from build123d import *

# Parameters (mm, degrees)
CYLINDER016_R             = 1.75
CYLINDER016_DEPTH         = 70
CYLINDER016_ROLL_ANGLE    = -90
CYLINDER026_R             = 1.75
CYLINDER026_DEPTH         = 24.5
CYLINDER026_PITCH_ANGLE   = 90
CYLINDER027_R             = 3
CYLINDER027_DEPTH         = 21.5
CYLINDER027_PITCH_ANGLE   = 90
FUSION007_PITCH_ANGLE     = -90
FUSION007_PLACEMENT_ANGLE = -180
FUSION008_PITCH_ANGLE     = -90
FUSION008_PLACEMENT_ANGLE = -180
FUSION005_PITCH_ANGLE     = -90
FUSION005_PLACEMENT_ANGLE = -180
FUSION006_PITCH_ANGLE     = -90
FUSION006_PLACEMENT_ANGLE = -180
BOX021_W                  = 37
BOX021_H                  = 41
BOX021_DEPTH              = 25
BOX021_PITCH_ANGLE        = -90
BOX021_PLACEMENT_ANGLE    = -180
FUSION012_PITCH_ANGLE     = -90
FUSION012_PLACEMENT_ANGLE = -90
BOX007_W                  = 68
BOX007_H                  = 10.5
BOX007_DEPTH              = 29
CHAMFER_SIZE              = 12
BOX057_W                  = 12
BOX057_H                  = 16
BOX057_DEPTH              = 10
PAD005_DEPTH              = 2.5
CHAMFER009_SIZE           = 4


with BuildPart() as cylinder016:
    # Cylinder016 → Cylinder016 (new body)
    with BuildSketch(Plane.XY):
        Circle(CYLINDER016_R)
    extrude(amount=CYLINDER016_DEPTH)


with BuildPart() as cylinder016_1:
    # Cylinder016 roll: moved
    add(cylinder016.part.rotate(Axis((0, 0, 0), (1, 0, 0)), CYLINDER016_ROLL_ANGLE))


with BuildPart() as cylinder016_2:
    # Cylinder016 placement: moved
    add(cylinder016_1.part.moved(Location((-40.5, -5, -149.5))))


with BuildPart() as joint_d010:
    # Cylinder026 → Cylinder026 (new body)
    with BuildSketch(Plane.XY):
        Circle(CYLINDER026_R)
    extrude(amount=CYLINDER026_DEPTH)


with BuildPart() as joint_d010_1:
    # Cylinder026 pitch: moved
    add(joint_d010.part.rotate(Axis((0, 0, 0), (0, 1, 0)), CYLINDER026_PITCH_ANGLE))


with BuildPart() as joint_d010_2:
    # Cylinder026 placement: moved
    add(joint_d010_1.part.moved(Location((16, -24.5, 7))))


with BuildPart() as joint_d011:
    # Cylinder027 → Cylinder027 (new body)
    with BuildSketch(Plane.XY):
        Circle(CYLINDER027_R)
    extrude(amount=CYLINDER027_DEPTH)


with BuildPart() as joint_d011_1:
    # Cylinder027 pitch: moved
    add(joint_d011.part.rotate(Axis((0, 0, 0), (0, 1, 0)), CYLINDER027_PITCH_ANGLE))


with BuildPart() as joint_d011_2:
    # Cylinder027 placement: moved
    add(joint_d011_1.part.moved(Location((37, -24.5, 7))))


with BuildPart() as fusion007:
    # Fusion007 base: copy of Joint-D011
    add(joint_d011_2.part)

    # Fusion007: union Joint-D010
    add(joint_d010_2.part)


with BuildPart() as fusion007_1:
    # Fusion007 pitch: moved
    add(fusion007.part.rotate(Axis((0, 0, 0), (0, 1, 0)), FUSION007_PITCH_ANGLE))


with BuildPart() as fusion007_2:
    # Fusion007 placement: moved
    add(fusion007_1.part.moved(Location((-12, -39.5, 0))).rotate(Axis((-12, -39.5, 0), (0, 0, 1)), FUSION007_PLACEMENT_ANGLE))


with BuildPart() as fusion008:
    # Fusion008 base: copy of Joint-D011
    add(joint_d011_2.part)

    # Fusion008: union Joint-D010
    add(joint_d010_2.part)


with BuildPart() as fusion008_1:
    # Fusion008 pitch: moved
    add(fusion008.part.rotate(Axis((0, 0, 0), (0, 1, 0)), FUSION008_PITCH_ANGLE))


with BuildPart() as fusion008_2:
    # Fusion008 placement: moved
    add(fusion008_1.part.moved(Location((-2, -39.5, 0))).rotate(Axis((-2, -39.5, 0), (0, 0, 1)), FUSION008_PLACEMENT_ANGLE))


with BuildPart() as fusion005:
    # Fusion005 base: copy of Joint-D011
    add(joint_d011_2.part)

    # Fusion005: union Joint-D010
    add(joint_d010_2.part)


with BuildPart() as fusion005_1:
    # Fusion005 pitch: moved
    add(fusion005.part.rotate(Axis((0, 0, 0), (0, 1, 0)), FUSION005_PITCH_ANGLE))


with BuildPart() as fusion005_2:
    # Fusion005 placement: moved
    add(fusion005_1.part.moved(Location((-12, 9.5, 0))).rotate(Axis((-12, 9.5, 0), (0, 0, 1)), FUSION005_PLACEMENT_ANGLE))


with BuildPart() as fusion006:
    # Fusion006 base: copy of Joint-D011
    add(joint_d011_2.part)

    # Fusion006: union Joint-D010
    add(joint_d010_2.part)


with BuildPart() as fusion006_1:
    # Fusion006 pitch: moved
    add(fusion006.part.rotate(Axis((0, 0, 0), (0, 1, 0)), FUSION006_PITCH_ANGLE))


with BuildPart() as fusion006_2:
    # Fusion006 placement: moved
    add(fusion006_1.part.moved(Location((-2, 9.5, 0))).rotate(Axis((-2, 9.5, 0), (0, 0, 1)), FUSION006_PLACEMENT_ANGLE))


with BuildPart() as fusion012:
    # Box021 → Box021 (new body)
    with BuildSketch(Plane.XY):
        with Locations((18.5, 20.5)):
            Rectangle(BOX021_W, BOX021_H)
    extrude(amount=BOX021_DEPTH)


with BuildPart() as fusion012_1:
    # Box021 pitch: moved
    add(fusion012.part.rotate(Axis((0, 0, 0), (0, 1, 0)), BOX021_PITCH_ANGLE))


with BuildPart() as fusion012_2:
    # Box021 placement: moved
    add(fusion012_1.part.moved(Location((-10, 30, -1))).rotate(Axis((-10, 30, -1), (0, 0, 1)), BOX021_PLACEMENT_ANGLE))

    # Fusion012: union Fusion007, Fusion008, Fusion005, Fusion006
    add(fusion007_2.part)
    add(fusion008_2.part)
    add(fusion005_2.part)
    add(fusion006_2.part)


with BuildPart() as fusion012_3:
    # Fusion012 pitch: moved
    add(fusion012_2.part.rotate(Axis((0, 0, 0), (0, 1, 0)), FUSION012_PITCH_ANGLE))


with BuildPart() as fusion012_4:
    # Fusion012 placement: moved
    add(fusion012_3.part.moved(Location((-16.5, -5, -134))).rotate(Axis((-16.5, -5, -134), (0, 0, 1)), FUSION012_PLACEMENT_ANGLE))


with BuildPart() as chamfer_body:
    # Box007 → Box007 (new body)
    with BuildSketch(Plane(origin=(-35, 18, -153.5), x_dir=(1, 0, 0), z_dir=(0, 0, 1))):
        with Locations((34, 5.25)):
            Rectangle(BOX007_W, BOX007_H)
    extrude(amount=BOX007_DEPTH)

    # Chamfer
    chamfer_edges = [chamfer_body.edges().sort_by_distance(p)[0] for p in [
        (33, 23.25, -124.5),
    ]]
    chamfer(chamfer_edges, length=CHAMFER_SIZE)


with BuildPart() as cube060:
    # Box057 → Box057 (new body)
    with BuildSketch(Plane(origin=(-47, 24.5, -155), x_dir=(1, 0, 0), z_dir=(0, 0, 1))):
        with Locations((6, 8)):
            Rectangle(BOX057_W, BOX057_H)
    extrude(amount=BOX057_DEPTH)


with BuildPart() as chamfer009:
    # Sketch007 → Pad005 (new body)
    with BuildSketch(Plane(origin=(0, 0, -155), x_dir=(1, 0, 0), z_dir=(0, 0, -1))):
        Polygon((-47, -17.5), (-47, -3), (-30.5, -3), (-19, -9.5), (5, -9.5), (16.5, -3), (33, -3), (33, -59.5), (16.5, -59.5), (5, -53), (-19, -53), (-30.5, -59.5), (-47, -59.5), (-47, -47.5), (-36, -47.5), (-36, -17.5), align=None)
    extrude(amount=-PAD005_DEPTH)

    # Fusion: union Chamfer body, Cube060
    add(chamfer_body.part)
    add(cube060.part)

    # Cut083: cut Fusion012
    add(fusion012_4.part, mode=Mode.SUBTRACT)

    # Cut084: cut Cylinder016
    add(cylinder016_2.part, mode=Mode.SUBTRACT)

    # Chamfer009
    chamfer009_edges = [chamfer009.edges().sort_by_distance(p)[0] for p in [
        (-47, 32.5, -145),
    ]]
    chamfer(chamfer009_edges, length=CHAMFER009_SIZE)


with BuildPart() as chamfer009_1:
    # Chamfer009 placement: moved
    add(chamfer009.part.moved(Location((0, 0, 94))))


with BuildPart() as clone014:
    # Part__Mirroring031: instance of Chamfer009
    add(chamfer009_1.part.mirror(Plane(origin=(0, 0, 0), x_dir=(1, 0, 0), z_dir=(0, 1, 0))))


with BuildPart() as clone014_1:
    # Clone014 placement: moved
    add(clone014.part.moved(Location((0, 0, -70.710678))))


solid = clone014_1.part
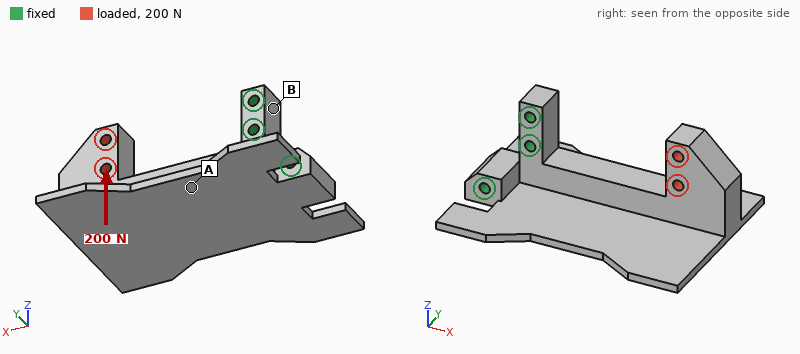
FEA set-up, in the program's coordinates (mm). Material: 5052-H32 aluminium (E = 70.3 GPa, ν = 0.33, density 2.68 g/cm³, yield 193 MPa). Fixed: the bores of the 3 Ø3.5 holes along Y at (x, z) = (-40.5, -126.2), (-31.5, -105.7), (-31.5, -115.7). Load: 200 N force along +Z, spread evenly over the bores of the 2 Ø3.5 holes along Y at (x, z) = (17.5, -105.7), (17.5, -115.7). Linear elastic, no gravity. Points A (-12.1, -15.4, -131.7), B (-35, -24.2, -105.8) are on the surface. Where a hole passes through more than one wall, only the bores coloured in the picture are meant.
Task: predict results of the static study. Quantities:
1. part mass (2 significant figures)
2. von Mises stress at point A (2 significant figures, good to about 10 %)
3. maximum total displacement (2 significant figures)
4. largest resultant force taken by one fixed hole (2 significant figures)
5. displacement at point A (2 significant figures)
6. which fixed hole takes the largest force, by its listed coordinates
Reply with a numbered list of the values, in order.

1. 57 g
2. 15 MPa
3. 0.14 mm
4. 730 N
5. 0.030 mm
6. (-31.5, -115.7)
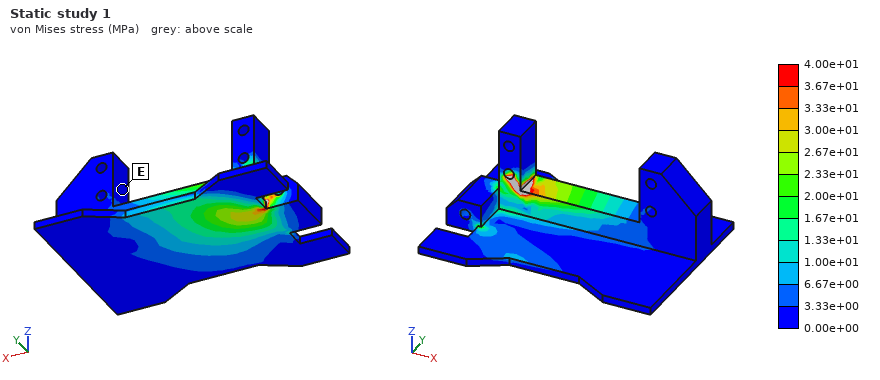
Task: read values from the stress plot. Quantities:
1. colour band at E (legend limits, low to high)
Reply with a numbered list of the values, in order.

1. 0.00e+00 to 3.33e+00 MPa
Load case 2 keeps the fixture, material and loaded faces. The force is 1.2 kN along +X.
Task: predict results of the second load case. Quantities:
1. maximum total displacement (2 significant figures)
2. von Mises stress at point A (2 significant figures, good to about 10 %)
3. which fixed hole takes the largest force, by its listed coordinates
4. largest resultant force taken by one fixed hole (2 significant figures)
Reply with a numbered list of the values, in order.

1. 0.40 mm
2. 44 MPa
3. (-31.5, -115.7)
4. 1.5 kN
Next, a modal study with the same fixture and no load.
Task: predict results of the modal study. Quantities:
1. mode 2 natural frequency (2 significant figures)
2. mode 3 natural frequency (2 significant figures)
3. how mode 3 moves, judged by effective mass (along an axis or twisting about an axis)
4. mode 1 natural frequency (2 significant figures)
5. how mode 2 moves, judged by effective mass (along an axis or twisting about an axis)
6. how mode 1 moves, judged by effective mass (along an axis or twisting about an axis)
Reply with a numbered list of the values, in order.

1. 1800 Hz
2. 2400 Hz
3. along Y
4. 1200 Hz
5. along Y
6. along Z
